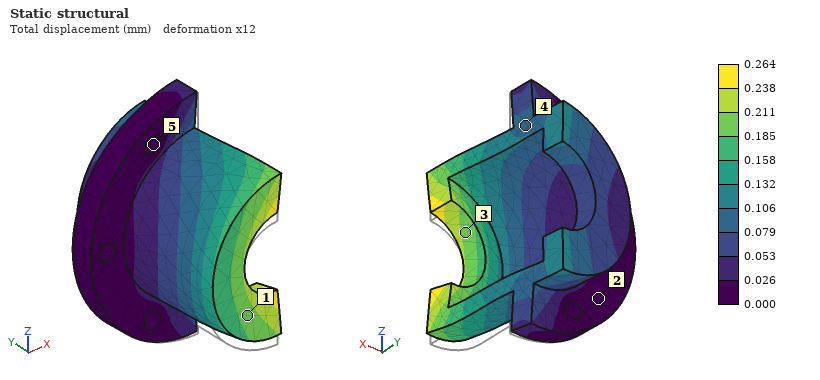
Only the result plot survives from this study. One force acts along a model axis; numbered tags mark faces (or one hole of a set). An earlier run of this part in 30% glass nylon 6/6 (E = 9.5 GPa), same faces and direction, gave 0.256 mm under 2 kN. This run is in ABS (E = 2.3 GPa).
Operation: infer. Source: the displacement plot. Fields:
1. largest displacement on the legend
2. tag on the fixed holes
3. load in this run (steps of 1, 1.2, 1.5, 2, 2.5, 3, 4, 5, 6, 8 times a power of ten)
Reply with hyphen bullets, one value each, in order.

- 0.264 mm
- 5
- 500 N
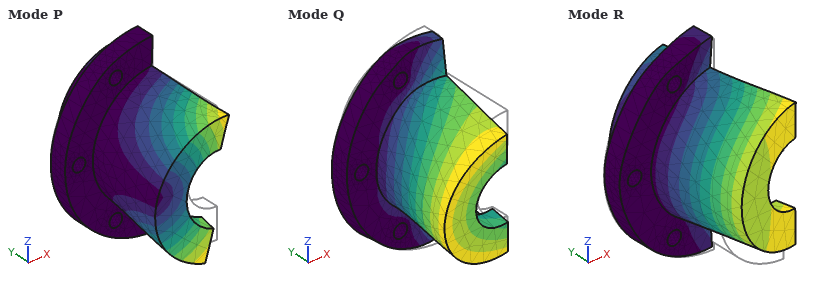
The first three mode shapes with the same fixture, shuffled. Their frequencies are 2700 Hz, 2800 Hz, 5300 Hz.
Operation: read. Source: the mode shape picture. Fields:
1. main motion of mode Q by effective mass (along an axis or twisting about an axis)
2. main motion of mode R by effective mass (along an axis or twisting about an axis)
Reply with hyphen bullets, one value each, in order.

- along Z
- along X
